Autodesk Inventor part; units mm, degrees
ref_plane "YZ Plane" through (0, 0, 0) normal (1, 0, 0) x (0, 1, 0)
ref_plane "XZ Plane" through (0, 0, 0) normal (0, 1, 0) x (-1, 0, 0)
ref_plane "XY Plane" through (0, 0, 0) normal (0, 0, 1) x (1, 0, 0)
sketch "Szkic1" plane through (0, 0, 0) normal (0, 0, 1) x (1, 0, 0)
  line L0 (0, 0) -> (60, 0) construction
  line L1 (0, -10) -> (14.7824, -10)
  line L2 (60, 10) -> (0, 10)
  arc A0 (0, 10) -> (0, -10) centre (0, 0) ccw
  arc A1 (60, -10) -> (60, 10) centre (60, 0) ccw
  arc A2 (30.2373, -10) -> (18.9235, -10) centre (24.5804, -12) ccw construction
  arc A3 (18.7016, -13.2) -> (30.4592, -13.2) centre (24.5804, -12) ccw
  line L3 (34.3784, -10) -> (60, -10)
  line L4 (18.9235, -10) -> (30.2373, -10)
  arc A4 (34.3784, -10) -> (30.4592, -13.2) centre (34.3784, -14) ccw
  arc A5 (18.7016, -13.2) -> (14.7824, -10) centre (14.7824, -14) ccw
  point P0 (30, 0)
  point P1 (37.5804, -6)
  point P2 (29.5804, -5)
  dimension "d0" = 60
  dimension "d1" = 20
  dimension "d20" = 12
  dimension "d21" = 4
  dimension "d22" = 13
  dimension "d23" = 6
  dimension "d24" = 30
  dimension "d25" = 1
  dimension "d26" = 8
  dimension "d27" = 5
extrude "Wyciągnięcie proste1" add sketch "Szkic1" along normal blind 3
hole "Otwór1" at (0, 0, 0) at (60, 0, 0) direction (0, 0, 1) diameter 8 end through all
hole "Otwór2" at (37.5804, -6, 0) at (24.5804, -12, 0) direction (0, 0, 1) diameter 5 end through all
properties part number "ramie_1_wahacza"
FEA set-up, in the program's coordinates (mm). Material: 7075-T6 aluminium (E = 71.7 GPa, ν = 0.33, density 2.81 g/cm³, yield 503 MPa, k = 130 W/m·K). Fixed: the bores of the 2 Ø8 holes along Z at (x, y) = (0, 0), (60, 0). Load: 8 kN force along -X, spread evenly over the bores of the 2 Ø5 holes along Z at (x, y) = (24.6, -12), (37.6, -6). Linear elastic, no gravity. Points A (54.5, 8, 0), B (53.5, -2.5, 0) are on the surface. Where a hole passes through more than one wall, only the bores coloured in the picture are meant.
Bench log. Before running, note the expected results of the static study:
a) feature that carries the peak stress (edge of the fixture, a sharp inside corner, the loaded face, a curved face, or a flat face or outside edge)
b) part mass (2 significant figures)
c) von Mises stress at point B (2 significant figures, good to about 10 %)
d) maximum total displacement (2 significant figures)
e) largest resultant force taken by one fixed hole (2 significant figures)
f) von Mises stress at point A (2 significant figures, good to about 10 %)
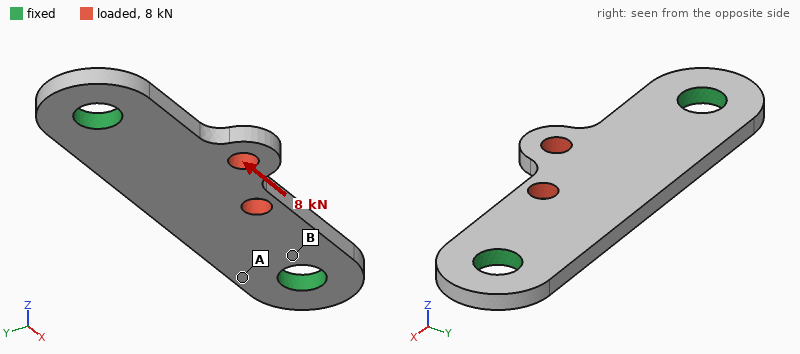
the loaded face
12 g
110 MPa
79 µm
4.3 kN
40 MPa
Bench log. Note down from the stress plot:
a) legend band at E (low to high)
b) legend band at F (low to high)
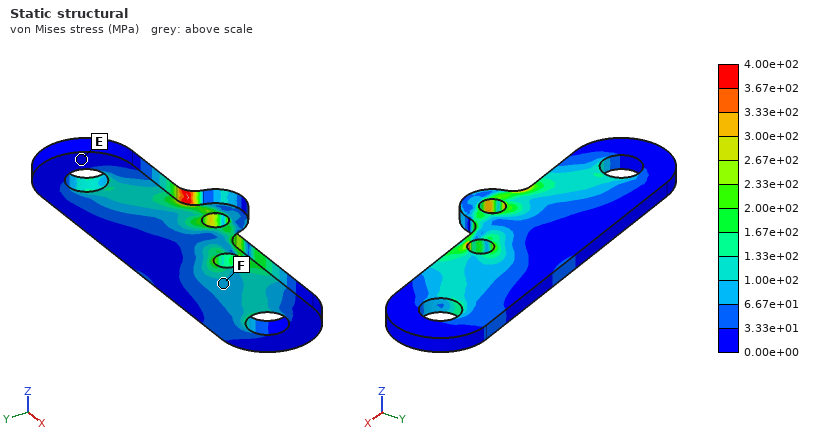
0.00e+00 to 3.33e+01 MPa
6.67e+01 to 1.00e+02 MPa
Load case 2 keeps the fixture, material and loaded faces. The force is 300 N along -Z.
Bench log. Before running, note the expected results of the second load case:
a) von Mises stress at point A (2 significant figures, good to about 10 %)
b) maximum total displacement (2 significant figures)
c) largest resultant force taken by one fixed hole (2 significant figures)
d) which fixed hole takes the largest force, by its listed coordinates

28 MPa
0.19 mm
160 N
(60, 0)
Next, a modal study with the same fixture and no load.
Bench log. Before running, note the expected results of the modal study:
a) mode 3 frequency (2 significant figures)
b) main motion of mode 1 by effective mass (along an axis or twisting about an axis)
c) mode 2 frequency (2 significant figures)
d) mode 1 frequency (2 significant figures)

13 kHz
along Z
7100 Hz
4800 Hz
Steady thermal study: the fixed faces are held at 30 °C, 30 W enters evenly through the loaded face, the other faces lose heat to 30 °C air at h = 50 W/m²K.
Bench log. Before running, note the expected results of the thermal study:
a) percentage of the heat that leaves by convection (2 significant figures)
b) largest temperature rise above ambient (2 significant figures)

11 %
63 K
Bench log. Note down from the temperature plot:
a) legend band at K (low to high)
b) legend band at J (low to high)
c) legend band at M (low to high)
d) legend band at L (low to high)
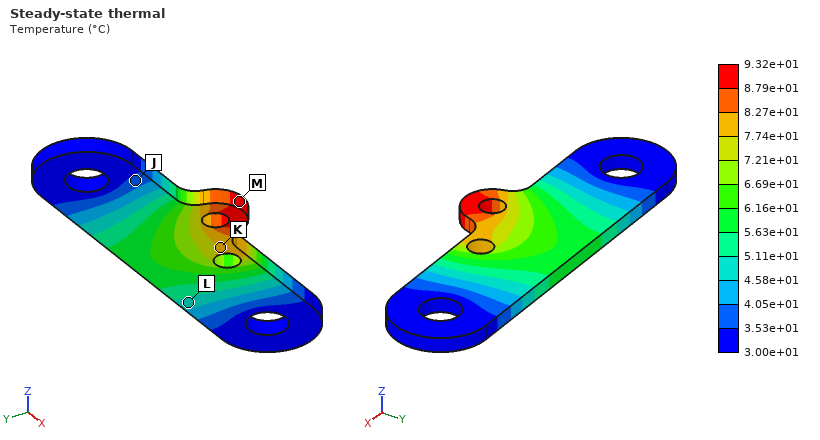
7.74e+01 to 8.27e+01 °C
3.53e+01 to 4.05e+01 °C
8.79e+01 to 9.32e+01 °C
4.58e+01 to 5.11e+01 °C
